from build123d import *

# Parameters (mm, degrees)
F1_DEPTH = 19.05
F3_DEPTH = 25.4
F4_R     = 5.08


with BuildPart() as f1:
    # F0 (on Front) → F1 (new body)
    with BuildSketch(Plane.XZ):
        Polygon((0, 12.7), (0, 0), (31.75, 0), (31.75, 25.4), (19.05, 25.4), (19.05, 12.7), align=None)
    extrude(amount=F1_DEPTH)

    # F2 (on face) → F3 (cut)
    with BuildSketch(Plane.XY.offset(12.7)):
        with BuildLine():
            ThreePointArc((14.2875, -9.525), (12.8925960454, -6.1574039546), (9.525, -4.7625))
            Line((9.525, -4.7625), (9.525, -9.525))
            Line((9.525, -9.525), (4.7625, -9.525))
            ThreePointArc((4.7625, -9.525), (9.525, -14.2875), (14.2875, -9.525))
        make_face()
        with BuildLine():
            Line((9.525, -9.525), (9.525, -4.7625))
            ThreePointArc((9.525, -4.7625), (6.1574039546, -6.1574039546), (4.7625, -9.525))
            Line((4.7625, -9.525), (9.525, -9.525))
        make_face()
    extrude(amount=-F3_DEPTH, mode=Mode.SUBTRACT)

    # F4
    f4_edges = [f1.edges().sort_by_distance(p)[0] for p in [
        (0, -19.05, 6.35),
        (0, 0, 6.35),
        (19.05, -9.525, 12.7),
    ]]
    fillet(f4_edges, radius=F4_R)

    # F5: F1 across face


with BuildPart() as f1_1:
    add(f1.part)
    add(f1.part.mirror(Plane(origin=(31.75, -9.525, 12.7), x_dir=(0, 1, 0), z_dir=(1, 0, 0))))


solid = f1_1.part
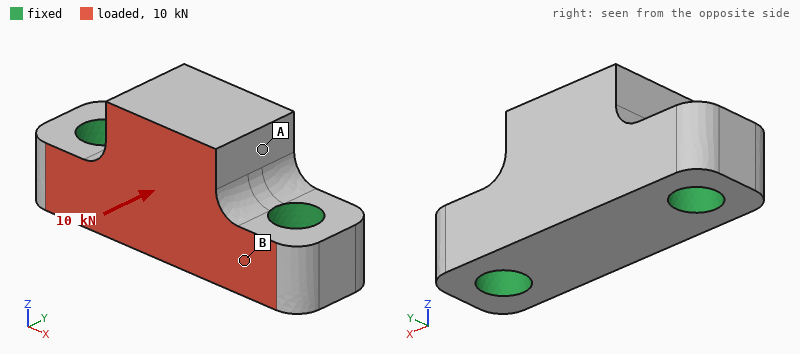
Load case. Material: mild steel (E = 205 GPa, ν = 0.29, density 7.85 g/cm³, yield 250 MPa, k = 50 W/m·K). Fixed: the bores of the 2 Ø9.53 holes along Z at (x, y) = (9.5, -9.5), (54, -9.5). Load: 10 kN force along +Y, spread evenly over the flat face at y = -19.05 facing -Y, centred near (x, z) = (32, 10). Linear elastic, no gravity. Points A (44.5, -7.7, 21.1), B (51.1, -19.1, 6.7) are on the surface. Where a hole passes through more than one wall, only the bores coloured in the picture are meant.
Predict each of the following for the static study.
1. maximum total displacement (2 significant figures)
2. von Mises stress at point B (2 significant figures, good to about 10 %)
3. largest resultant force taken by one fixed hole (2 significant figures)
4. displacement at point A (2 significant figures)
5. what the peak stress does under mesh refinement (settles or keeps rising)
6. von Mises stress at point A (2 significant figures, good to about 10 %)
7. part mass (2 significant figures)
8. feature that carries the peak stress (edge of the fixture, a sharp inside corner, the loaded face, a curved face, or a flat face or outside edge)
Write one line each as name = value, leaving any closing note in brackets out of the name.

maximum total displacement = 9.9 µm
von Mises stress at point B = 36 MPa
largest resultant force taken by one fixed hole = 5.0 kN
displacement at point A = 7.0 µm
what the peak stress does under mesh refinement = keeps rising
von Mises stress at point A = 15 MPa
part mass = 150 g
feature that carries the peak stress = edge of the fixture
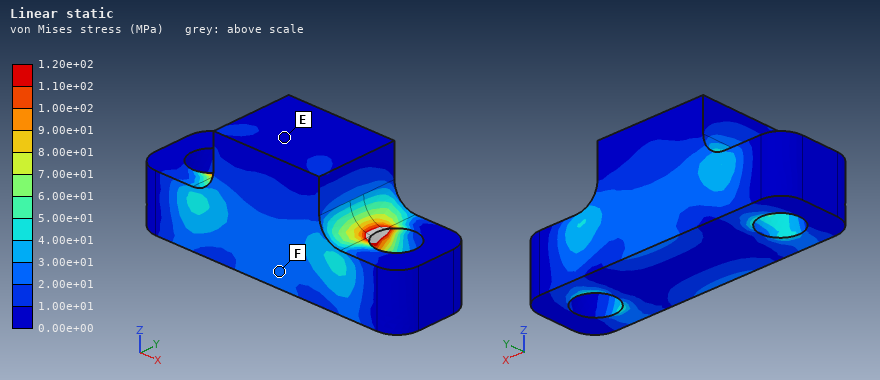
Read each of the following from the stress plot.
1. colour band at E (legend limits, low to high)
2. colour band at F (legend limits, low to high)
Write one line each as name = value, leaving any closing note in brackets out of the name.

colour band at E = 0.00e+00 to 1.00e+01 MPa
colour band at F = 2.00e+01 to 3.00e+01 MPa
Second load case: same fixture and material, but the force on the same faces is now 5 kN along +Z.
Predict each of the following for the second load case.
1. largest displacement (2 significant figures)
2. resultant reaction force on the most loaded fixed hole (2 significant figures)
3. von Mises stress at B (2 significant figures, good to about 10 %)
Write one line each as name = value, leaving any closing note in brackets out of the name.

largest displacement = 6.7 µm
resultant reaction force on the most loaded fixed hole = 2.6 kN
von Mises stress at B = 30 MPa
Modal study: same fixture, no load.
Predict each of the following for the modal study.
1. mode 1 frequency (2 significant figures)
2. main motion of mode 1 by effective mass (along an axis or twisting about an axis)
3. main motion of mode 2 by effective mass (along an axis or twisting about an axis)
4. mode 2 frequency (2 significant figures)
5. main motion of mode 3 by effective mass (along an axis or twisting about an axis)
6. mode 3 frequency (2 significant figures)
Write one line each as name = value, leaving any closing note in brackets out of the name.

mode 1 frequency = 16 kHz
main motion of mode 1 by effective mass = along Y
main motion of mode 2 by effective mass = along Z
mode 2 frequency = 26 kHz
main motion of mode 3 by effective mass = along Y
mode 3 frequency = 31 kHz
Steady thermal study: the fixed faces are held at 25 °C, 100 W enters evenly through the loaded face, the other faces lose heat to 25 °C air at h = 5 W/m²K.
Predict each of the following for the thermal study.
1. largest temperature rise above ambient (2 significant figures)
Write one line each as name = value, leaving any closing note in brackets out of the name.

largest temperature rise above ambient = 52 K
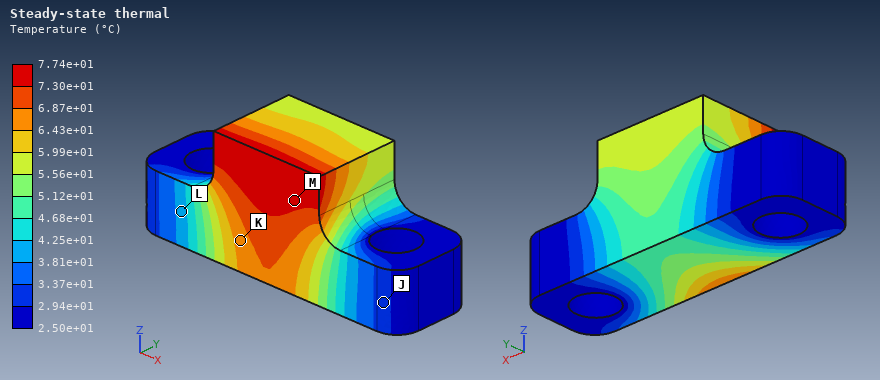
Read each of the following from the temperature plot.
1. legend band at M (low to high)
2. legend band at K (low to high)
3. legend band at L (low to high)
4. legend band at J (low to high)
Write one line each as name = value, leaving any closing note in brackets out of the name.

legend band at M = 7.30e+01 to 7.74e+01 °C
legend band at K = 6.43e+01 to 6.87e+01 °C
legend band at L = 3.81e+01 to 4.25e+01 °C
legend band at J = 2.94e+01 to 3.37e+01 °C
